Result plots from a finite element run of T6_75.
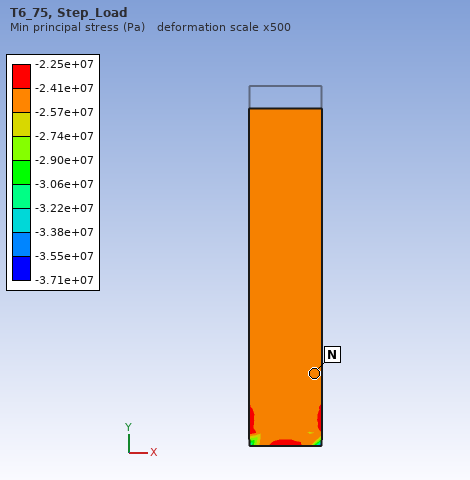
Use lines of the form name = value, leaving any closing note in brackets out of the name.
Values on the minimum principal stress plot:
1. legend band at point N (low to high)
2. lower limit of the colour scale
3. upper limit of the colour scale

legend band at point N = -2.57e+07 to -2.41e+07 Pa
lower limit of the colour scale = -3.71e+07 Pa
upper limit of the colour scale = -2.25e+07 Pa
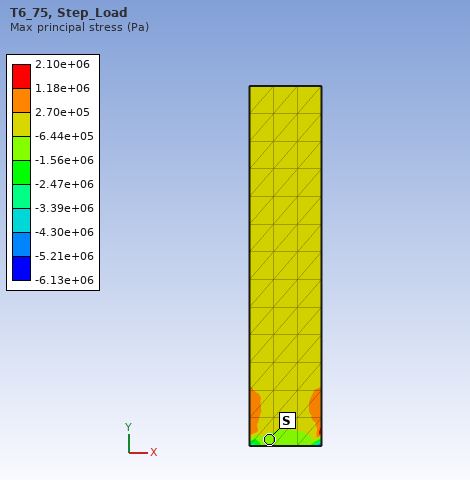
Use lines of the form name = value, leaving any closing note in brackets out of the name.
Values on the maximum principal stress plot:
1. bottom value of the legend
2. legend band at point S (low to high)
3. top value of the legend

bottom value of the legend = -6.13e+06 Pa
legend band at point S = -1.56e+06 to -6.44e+05 Pa
top value of the legend = 2.10e+06 Pa
